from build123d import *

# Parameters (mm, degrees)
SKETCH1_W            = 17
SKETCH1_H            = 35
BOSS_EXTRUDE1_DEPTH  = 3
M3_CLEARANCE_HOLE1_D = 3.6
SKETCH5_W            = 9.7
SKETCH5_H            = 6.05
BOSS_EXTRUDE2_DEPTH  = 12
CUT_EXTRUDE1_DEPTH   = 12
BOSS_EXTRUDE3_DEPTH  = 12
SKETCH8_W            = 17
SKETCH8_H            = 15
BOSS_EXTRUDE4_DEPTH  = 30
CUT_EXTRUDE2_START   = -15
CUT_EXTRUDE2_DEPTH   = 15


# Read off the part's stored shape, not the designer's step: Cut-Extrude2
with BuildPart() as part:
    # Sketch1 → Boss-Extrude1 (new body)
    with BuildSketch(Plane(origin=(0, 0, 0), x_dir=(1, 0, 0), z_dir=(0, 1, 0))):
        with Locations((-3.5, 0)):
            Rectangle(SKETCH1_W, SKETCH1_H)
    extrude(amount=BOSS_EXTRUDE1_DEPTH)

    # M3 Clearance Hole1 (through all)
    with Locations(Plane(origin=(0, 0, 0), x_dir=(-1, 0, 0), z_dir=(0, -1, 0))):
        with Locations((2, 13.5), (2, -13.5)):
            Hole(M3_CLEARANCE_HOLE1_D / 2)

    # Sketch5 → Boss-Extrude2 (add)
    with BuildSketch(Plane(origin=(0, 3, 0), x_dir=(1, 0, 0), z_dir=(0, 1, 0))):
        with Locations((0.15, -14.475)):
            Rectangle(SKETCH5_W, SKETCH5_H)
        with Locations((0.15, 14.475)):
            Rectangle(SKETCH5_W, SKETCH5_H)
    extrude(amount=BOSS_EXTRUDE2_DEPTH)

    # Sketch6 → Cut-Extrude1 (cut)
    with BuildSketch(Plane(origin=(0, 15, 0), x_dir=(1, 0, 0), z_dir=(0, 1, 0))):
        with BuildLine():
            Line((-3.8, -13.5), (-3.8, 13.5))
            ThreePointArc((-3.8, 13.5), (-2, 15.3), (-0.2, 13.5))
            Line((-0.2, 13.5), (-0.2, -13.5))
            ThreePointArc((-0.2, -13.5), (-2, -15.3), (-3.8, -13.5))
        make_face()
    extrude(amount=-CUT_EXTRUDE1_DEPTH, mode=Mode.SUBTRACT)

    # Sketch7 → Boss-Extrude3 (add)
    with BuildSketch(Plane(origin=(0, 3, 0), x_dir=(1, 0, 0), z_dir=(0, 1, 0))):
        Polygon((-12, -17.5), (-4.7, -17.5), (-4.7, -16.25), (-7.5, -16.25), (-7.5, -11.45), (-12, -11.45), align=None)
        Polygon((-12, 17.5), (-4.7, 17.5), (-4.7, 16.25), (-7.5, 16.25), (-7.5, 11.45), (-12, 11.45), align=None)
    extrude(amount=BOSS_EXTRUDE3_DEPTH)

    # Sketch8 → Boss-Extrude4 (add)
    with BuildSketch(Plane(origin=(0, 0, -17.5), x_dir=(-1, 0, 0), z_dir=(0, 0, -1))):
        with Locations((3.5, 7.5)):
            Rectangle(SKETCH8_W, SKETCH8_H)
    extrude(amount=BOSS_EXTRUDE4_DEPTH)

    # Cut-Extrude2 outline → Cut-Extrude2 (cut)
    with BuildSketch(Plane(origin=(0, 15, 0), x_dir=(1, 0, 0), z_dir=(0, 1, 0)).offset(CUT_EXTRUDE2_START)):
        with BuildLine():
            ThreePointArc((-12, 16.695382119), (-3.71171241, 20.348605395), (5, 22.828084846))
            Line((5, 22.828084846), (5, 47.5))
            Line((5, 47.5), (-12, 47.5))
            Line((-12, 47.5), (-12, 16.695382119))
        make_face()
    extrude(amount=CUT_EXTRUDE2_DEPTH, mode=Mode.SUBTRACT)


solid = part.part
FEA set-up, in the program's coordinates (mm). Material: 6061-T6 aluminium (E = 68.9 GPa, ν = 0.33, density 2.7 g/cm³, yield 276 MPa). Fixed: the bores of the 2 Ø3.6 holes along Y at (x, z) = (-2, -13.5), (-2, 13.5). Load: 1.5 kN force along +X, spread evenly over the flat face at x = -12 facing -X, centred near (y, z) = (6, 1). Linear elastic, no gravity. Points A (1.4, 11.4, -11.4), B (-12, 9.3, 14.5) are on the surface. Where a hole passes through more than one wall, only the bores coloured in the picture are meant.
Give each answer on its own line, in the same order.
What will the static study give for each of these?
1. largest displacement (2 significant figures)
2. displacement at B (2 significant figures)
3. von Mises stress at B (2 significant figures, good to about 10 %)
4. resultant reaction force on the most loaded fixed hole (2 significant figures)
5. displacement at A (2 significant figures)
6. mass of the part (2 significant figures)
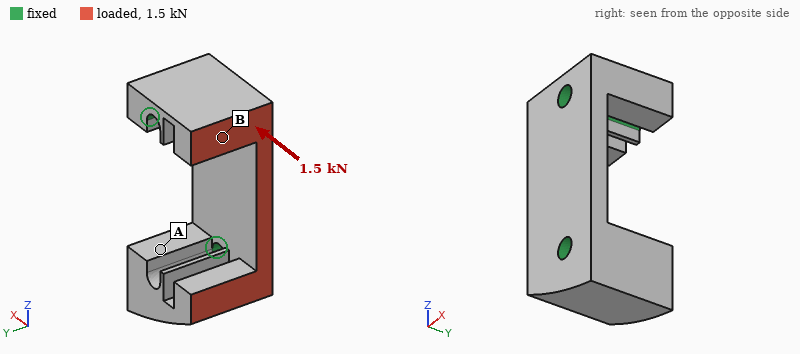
39 µm
10 µm
27 MPa
780 N
16 µm
12 g
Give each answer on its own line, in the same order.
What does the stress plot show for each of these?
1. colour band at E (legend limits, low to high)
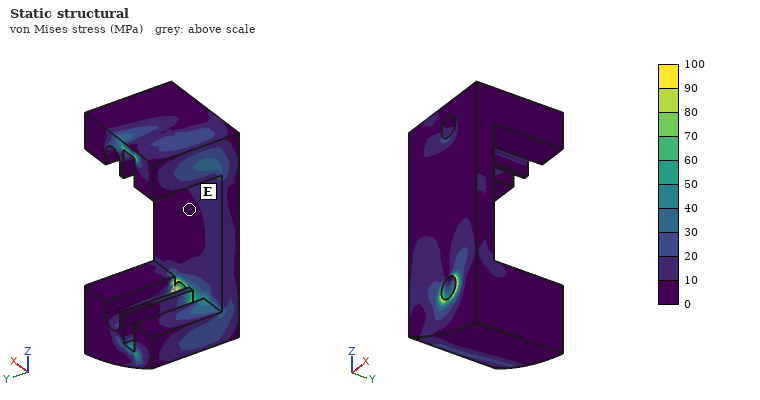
0 to 10 MPa
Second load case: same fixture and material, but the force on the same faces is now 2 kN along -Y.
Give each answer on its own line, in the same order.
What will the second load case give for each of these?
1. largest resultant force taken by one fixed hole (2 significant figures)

1.1 kN
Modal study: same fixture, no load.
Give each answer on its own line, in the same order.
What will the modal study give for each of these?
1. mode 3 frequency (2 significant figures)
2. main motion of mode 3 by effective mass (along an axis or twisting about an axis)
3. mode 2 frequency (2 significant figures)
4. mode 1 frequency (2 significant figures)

20 kHz
along Y
12 kHz
11 kHz
